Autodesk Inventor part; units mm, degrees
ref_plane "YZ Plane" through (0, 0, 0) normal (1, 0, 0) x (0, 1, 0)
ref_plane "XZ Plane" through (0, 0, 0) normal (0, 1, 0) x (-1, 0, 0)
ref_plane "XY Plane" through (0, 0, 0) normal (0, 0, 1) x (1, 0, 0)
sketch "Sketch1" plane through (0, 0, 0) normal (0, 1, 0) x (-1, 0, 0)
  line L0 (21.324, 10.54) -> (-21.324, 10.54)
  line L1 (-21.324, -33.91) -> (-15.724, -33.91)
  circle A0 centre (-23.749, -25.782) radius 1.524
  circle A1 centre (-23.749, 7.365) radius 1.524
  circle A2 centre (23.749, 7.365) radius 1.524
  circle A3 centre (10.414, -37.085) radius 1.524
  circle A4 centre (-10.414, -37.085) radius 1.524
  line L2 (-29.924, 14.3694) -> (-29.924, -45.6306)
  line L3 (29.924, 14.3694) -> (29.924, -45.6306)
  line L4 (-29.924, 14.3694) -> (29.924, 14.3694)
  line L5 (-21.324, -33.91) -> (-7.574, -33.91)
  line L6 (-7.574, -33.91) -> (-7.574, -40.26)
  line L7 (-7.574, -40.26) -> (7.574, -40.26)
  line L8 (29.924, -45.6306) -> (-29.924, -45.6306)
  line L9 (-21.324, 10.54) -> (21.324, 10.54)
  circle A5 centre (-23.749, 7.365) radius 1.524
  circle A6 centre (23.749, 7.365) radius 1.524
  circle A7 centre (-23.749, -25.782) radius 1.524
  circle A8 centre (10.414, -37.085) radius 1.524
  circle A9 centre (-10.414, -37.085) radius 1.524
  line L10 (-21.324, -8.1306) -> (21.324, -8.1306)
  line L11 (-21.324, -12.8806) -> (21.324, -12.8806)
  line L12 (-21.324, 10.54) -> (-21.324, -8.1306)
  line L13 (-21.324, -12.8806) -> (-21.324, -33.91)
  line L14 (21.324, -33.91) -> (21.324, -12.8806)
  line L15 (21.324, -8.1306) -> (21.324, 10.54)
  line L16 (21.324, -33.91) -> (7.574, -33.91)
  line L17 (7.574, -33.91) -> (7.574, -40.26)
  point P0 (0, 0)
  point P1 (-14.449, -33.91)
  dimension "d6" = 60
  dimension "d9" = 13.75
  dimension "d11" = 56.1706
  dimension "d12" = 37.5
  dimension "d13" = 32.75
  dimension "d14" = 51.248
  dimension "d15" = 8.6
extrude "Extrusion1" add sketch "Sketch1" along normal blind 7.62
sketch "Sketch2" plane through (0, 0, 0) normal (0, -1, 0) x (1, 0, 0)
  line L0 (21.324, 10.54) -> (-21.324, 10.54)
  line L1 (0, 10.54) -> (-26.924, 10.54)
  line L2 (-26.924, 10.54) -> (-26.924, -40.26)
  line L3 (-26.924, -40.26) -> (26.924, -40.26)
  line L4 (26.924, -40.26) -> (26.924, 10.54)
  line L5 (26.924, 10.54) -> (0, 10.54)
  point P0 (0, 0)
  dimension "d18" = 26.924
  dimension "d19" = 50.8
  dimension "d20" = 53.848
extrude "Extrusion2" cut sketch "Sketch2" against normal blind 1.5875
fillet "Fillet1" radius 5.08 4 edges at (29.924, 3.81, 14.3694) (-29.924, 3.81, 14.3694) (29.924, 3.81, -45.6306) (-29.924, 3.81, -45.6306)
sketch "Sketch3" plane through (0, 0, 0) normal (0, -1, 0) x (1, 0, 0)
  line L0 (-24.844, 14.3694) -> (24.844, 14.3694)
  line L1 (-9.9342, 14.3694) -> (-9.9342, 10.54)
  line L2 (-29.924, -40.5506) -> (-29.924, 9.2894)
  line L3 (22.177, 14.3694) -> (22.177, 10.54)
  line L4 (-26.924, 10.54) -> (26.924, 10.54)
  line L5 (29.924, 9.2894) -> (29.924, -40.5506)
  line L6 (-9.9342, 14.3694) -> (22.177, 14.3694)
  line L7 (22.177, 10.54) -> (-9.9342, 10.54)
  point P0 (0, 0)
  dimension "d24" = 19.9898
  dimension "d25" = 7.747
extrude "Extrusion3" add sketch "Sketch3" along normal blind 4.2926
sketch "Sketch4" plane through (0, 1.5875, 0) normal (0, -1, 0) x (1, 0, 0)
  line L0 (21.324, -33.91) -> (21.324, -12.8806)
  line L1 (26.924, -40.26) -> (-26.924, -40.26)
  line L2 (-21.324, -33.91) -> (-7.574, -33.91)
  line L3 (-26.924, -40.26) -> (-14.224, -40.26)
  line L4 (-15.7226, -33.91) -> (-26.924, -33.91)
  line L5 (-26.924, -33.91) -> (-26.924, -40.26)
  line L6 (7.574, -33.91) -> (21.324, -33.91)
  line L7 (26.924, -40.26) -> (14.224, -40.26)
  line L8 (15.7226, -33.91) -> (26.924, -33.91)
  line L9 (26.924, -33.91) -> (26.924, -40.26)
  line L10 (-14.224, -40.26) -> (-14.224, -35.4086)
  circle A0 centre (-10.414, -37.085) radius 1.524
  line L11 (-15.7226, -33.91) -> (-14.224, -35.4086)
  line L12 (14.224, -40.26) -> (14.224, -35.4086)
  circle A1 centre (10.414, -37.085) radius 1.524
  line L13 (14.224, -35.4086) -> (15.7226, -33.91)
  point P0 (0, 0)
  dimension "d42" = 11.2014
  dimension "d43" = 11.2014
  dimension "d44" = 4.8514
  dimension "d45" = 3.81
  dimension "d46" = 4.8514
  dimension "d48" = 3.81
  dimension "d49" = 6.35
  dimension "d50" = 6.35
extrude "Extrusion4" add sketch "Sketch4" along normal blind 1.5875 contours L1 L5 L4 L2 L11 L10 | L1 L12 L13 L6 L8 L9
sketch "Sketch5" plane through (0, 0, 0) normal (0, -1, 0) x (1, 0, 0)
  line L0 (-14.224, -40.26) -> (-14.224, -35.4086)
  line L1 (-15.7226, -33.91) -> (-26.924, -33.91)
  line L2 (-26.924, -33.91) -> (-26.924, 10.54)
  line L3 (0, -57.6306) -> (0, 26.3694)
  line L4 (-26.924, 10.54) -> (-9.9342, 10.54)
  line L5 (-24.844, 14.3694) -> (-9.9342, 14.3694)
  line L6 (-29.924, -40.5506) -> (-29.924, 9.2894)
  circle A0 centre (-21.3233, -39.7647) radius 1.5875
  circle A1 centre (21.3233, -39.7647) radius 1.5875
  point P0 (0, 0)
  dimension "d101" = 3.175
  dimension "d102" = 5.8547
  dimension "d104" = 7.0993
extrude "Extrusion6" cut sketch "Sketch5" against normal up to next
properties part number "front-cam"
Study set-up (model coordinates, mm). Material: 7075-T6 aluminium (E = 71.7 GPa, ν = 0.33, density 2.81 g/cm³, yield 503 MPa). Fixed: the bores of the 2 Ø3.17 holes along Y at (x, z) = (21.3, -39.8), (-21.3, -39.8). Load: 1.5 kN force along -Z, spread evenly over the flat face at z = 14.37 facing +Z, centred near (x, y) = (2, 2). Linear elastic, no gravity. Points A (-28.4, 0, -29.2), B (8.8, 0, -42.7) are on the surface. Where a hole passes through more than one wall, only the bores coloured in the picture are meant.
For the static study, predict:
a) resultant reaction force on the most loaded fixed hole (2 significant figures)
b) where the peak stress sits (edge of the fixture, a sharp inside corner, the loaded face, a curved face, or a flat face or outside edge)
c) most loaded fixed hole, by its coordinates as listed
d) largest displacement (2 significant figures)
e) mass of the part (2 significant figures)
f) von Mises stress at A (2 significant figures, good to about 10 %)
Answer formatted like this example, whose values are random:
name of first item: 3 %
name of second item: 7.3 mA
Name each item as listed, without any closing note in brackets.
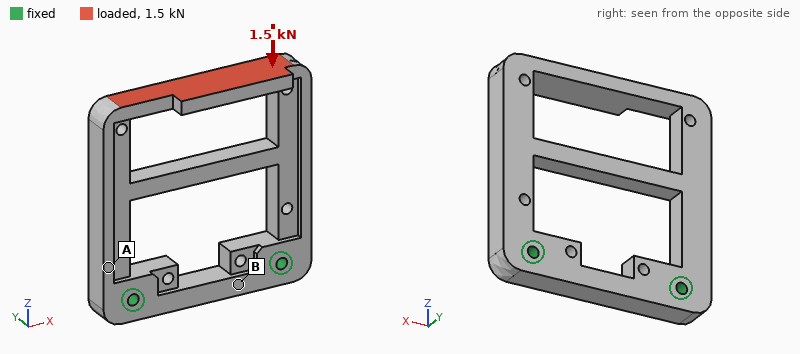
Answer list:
resultant reaction force on the most loaded fixed hole: 800 N
where the peak stress sits: a curved face
most loaded fixed hole, by its coordinates as listed: (21.3, -39.8)
largest displacement: 0.32 mm
mass of the part: 35 g
von Mises stress at A: 37 MPa
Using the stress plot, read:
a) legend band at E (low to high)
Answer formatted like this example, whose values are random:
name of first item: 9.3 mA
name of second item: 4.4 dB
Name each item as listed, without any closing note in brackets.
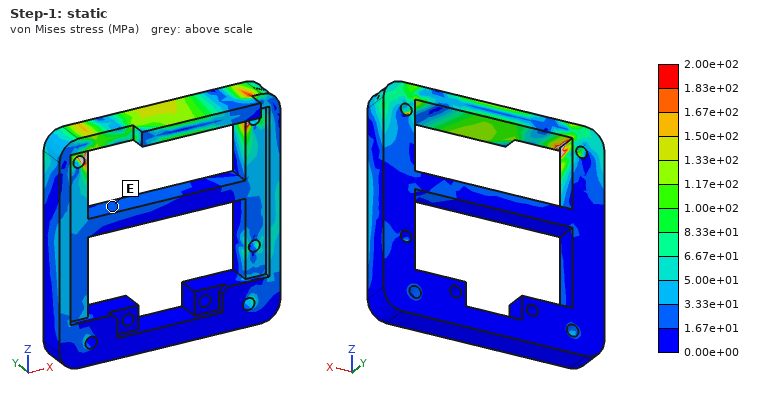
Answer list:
legend band at E: 1.67e+01 to 3.33e+01 MPa
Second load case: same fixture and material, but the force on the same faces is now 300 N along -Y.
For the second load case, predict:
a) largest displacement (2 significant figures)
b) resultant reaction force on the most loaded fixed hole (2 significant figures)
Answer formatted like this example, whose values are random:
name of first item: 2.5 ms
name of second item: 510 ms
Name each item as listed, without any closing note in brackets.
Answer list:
largest displacement: 0.54 mm
resultant reaction force on the most loaded fixed hole: 160 N
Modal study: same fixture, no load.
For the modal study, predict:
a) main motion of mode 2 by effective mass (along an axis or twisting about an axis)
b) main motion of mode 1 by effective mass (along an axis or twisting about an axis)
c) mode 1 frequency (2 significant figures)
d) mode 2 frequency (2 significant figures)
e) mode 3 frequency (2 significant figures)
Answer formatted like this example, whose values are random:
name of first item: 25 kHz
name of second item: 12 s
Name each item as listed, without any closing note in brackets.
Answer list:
main motion of mode 2 by effective mass: along X
main motion of mode 1 by effective mass: along Y
mode 1 frequency: 1300 Hz
mode 2 frequency: 2200 Hz
mode 3 frequency: 2600 Hz
